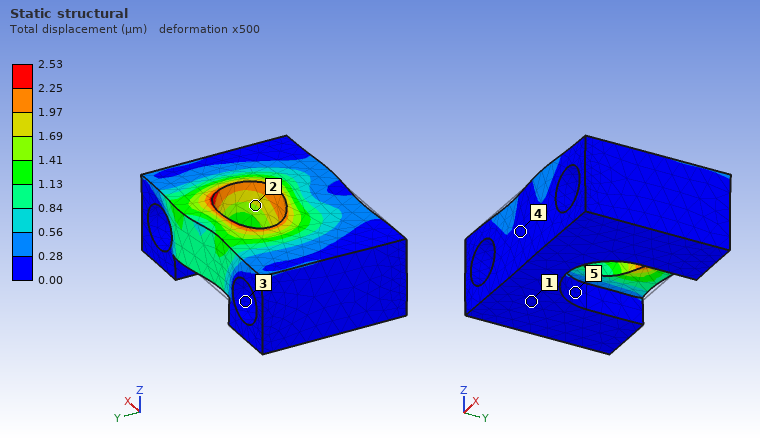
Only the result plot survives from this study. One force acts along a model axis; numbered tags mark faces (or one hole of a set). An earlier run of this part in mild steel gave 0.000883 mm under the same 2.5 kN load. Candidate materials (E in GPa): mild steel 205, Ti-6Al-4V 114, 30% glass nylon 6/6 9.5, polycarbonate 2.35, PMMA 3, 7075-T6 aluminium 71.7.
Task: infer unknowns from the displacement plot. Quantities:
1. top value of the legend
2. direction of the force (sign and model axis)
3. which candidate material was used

2.53 µm
+X
7075-T6 aluminium
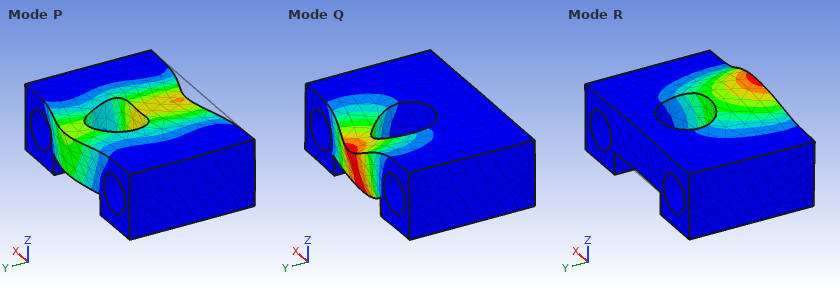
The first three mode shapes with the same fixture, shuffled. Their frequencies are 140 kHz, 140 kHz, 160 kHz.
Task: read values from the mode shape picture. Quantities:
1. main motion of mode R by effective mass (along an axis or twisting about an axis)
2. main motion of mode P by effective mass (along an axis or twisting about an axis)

along Z
along Y
